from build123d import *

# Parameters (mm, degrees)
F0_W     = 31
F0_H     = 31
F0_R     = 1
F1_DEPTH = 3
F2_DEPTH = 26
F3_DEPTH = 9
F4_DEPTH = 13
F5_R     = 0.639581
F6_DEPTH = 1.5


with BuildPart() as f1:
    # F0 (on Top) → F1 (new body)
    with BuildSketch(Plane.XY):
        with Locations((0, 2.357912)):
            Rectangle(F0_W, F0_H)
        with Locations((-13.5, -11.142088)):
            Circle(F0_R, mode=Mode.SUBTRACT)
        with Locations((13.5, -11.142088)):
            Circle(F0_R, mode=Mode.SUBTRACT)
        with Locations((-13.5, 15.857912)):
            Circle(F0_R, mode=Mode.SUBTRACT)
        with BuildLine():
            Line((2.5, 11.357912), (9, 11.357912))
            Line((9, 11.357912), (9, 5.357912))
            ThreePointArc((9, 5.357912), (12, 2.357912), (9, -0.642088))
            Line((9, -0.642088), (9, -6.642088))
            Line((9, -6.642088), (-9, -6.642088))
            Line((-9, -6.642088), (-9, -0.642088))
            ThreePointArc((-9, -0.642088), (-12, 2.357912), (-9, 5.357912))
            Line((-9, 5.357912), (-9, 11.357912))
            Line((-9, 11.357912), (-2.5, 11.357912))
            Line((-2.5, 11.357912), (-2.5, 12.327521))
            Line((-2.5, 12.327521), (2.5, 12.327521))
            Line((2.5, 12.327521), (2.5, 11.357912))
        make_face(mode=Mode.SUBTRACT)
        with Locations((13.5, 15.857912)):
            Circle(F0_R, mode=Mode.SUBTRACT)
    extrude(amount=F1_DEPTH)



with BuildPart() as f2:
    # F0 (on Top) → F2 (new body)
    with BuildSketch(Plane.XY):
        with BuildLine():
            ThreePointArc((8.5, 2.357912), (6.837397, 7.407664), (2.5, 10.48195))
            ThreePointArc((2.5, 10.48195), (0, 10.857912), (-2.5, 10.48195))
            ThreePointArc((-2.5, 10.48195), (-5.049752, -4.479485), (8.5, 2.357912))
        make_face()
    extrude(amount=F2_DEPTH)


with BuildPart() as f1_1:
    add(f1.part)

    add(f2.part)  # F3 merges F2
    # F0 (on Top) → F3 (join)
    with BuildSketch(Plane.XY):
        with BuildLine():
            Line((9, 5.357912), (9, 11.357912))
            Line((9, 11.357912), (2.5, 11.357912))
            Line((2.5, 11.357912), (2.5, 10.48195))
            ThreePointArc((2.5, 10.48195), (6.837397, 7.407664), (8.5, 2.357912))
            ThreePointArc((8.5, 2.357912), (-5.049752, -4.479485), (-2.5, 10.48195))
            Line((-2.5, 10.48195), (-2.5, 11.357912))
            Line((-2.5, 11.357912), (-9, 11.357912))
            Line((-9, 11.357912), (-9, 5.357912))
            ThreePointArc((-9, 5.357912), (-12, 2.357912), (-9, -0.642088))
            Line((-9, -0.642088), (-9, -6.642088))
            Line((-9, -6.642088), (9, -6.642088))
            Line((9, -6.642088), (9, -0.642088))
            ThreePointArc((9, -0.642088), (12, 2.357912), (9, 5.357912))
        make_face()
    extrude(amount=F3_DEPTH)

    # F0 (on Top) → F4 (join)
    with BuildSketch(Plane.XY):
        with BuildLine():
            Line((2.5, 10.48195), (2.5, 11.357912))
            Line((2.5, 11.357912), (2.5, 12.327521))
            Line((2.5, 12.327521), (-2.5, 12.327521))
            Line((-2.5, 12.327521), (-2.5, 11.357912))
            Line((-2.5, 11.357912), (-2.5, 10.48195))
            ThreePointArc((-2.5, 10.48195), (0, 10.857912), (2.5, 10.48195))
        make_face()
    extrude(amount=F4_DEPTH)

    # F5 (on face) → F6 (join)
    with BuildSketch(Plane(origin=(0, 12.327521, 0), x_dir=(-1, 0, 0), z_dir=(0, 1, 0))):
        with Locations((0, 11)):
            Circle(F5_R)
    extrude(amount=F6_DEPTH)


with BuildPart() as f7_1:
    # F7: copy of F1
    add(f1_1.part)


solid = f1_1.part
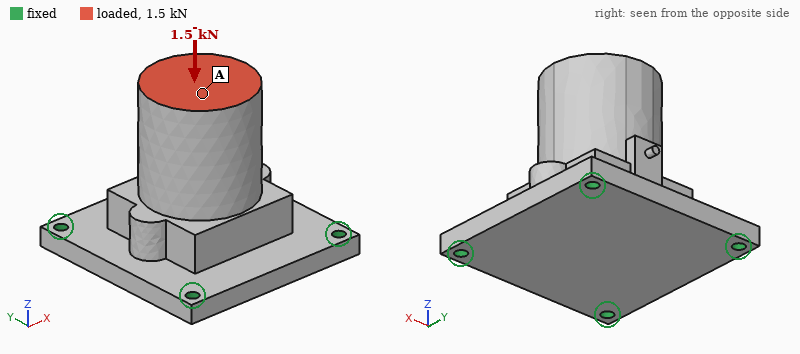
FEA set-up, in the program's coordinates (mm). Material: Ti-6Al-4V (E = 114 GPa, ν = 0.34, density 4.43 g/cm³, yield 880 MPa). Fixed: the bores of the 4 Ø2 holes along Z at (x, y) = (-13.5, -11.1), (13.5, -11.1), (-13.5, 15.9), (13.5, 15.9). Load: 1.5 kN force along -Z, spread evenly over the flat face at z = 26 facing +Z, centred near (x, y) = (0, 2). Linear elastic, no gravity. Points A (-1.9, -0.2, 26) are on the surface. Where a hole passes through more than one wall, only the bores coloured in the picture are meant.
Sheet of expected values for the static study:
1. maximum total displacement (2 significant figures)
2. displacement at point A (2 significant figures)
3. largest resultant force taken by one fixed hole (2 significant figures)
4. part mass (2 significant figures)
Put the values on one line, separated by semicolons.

14 µm; 14 µm; 400 N; 39 g
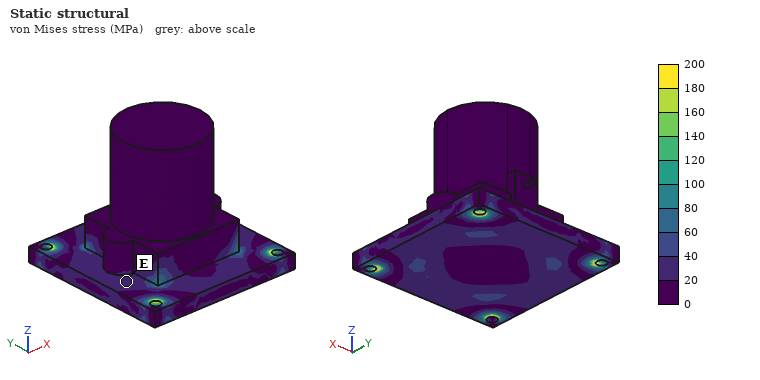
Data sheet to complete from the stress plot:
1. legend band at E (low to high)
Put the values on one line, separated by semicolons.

20 to 40 MPa
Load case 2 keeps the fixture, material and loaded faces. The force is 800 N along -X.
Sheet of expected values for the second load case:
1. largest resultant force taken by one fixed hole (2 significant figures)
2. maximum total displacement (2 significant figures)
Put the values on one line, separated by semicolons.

480 N; 41 µm
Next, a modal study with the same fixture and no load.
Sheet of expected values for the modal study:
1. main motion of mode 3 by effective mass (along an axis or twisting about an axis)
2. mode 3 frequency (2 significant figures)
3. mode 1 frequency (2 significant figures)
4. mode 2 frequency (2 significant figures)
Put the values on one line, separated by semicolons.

along Z; 9000 Hz; 7400 Hz; 7500 Hz
